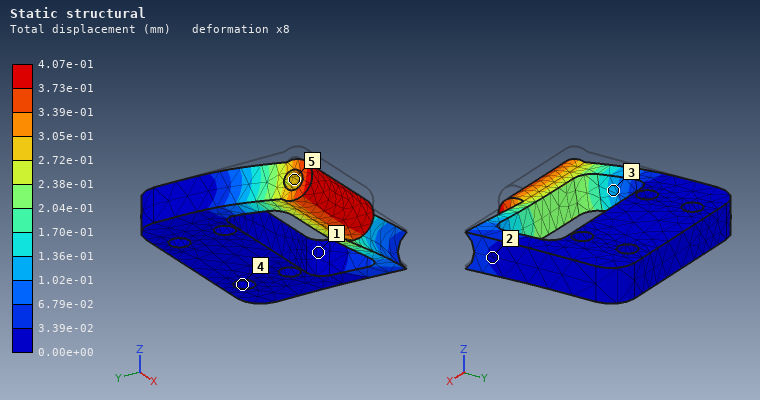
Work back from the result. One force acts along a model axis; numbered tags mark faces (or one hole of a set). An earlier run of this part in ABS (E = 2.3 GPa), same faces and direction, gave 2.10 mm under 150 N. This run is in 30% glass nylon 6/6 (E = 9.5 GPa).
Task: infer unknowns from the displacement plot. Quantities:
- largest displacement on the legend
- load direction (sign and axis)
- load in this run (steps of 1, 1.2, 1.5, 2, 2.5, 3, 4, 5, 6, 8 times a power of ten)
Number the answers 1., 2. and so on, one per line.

1. 4.07e-01 mm
2. -Z
3. 120 N
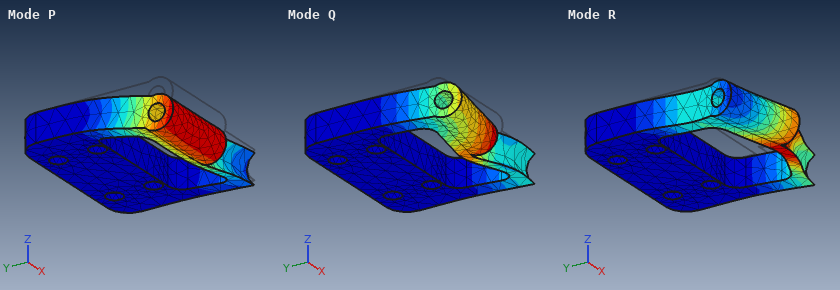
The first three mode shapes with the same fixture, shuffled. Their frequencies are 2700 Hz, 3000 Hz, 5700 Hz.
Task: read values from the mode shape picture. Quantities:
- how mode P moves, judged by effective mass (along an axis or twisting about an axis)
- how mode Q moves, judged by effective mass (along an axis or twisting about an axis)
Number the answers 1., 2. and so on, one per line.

1. along Z
2. along X
